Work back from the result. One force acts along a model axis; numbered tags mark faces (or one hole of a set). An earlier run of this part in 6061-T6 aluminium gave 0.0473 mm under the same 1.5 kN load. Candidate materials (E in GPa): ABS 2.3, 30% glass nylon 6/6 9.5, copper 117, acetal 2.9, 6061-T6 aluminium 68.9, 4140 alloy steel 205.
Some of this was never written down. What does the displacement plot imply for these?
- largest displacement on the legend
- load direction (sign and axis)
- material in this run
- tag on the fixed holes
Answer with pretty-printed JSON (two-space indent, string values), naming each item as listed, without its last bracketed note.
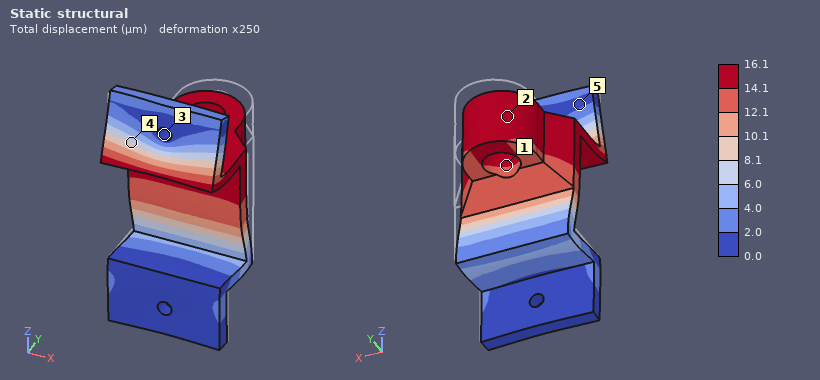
{
  "largest displacement on the legend": "16.1 µm",
  "load direction": "-Y",
  "material in this run": "4140 alloy steel",
  "tag on the fixed holes": "3"
}
